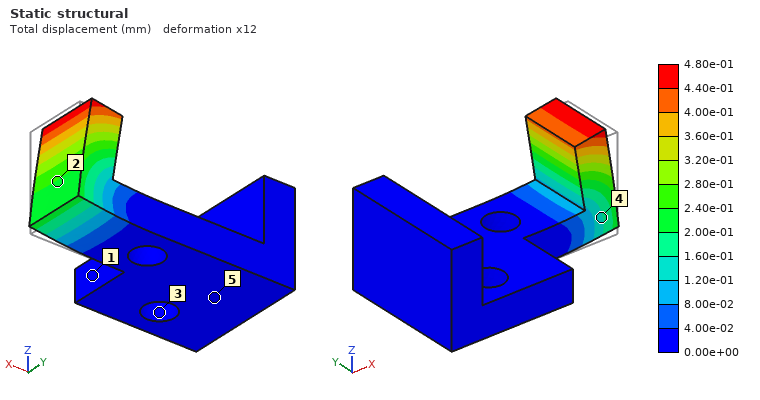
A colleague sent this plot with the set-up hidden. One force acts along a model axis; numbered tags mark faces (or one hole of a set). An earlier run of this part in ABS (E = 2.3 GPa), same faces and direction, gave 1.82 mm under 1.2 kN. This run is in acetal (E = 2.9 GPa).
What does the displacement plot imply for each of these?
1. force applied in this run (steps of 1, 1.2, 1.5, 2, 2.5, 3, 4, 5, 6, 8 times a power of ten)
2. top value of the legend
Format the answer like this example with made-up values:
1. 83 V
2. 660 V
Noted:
1. 400 N
2. 4.80e-01 mm
